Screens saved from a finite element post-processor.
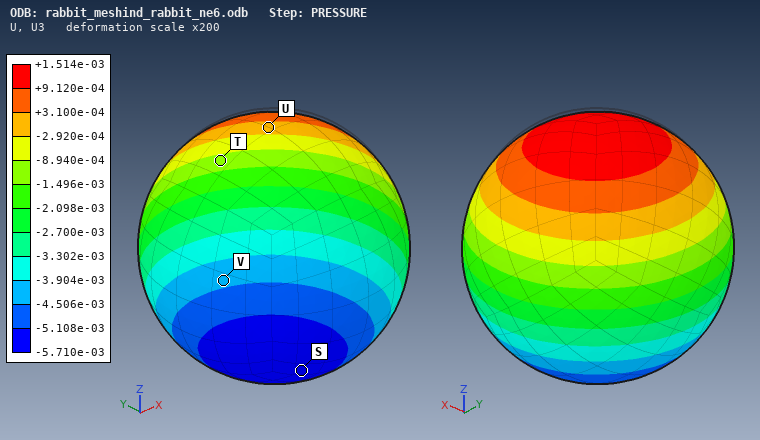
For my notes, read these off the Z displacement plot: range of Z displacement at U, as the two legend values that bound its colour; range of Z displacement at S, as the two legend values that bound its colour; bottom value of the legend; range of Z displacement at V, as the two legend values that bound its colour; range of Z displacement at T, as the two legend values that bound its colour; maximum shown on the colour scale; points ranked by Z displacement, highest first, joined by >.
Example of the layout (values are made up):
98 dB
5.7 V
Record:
-2.920e-04 to +3.100e-04
-5.710e-03 to -5.108e-03
-5.710e-03
-4.506e-03 to -3.904e-03
-1.496e-03 to -8.940e-04
+1.514e-03
U > T > V > S
